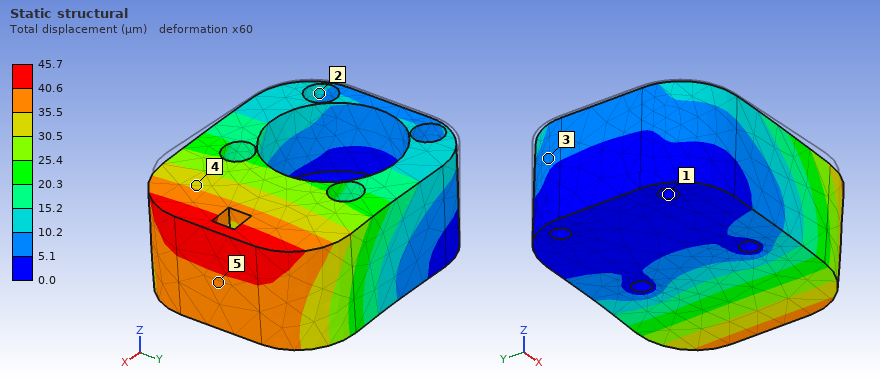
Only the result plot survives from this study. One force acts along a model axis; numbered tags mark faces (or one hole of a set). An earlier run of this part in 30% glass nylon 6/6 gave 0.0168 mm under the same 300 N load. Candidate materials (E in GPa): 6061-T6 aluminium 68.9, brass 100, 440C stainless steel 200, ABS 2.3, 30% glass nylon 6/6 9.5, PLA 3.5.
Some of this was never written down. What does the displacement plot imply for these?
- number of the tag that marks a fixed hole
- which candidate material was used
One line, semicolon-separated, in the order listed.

1; PLA
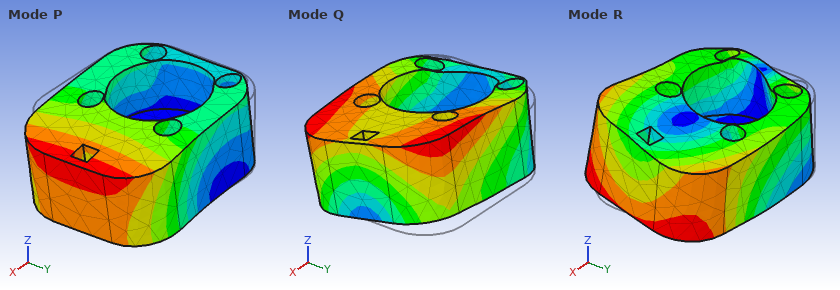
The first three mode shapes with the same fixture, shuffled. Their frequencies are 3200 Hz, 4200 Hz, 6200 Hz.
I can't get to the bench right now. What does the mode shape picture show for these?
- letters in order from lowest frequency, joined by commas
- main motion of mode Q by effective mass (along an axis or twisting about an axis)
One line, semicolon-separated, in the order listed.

P, Q, R; along Y
